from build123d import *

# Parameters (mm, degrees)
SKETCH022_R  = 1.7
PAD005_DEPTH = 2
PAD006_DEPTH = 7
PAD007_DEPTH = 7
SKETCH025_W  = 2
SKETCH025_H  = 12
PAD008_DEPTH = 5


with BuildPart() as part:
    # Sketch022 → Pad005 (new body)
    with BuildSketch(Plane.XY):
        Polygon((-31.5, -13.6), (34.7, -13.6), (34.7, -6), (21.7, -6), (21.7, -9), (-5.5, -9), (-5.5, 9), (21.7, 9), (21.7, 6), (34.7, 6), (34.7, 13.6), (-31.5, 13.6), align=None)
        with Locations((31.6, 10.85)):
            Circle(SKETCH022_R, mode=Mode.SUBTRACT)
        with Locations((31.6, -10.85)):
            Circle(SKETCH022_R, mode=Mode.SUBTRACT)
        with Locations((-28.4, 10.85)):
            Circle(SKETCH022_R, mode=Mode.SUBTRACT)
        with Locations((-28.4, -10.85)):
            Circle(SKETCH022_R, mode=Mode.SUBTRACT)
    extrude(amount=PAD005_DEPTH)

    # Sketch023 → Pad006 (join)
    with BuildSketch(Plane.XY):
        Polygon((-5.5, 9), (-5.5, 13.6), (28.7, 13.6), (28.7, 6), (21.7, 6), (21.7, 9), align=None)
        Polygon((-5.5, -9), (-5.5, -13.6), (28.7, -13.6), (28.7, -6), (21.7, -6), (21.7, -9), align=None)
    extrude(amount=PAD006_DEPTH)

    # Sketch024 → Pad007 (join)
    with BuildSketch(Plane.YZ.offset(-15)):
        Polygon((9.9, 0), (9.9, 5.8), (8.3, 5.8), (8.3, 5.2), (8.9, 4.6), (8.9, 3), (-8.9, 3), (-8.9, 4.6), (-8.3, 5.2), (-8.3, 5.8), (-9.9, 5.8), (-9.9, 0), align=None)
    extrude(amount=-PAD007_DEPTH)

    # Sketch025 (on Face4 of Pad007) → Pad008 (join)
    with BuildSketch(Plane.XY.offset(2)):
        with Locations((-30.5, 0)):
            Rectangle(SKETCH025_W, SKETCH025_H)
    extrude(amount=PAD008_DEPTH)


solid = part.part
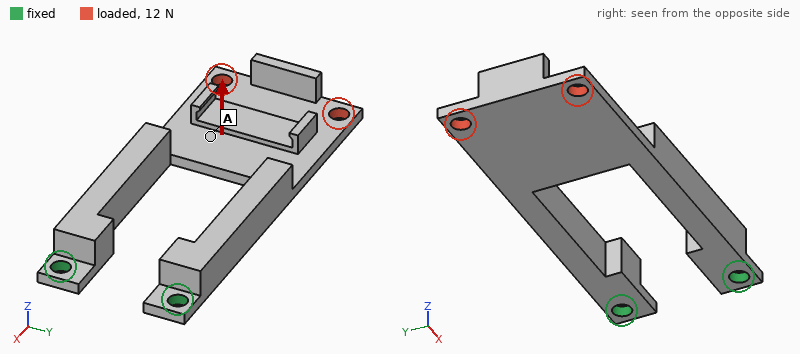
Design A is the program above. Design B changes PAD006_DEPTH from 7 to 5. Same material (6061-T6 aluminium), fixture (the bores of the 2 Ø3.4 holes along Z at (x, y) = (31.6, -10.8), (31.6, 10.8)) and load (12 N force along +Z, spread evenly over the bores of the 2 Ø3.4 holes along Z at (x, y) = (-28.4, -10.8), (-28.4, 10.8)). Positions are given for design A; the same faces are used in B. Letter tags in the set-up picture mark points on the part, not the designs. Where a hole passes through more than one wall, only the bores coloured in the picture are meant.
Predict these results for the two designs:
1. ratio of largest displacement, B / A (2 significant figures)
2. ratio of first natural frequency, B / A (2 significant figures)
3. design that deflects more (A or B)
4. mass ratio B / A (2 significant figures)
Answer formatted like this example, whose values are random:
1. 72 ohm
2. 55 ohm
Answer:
1. 1.2
2. 0.94
3. B
4. 0.84
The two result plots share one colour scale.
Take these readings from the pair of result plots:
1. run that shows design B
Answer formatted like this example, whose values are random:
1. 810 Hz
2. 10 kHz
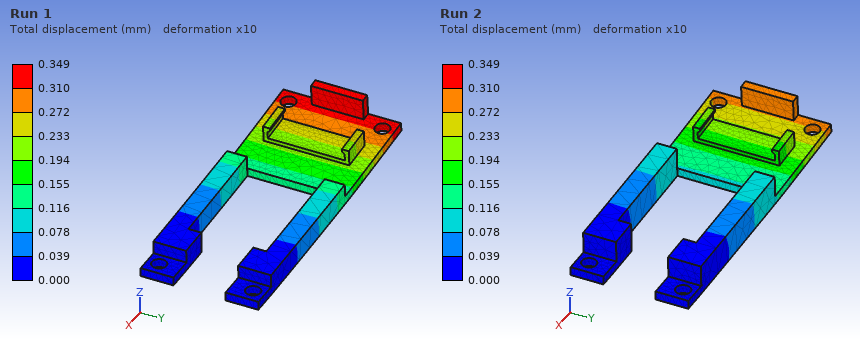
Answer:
1. Run 1
